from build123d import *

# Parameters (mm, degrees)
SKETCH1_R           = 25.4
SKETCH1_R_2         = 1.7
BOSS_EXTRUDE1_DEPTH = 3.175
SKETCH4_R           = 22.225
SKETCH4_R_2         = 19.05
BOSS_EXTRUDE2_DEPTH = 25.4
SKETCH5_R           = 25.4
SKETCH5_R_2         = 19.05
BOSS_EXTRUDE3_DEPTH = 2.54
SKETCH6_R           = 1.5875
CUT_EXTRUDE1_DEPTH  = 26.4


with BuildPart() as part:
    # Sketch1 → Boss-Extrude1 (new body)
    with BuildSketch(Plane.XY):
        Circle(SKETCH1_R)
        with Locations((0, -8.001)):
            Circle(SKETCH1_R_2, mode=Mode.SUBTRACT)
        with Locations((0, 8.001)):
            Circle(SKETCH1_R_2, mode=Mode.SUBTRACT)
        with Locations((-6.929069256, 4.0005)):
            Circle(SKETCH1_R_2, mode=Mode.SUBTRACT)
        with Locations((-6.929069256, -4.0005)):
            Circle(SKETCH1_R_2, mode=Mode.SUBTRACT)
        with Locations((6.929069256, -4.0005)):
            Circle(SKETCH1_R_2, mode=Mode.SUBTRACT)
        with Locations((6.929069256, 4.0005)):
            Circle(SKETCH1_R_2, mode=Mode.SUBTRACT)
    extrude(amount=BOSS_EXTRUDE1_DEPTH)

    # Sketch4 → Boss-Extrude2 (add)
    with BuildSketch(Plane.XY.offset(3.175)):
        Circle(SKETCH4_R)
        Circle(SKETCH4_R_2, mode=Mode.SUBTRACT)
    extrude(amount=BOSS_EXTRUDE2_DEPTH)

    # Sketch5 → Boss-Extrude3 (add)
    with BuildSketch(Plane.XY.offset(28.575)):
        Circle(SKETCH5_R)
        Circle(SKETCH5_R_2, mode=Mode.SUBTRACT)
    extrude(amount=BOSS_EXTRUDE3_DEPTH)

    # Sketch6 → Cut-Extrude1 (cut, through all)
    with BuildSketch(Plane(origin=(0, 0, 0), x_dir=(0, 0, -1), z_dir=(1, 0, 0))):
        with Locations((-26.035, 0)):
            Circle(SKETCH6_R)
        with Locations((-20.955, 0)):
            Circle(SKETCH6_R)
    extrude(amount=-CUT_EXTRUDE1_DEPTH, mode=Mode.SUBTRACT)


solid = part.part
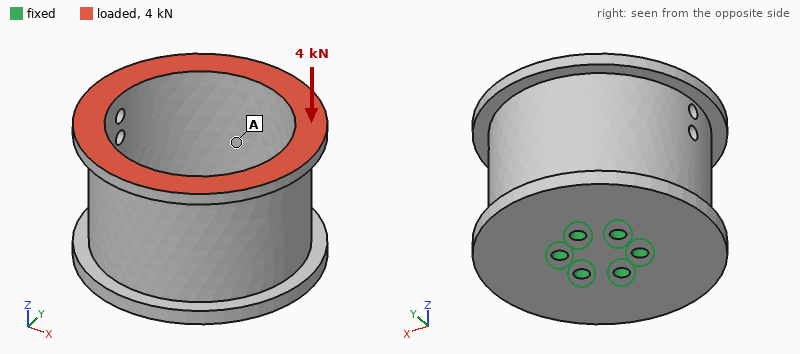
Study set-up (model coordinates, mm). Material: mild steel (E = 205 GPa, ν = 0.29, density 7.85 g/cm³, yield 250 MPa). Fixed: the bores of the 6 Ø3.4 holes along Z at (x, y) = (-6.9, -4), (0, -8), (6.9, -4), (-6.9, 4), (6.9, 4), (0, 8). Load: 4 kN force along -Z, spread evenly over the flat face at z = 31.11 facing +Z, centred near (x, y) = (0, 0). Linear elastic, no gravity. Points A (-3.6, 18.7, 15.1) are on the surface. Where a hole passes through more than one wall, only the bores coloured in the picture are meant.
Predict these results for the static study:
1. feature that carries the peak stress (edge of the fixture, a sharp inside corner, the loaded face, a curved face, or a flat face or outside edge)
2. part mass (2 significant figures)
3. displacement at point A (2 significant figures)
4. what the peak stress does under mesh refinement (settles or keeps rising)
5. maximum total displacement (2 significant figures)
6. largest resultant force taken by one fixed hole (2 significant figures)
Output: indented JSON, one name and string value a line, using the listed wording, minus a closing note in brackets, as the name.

{
  "feature that carries the peak stress": "edge of the fixture",
  "part mass": "150 g",
  "displacement at point A": "17 µm",
  "what the peak stress does under mesh refinement": "keeps rising",
  "maximum total displacement": "20 µm",
  "largest resultant force taken by one fixed hole": "700 N"
}
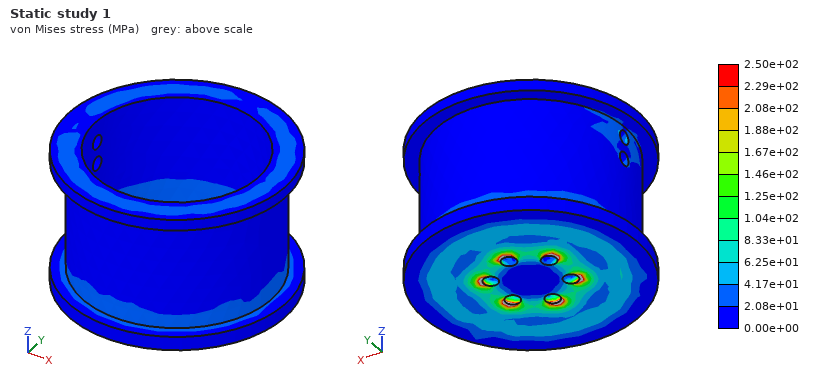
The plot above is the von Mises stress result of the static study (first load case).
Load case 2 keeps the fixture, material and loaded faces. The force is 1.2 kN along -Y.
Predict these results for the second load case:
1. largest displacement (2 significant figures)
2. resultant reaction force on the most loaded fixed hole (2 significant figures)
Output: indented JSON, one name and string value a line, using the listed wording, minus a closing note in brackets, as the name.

{
  "largest displacement": "51 µm",
  "resultant reaction force on the most loaded fixed hole": "810 N"
}
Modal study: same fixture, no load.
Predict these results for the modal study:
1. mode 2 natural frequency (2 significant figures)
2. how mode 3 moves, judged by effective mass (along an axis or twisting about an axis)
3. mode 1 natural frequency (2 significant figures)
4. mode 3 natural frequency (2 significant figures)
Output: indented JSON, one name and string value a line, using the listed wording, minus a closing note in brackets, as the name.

{
  "mode 2 natural frequency": "3300 Hz",
  "how mode 3 moves, judged by effective mass": "along Z",
  "mode 1 natural frequency": "3300 Hz",
  "mode 3 natural frequency": "6900 Hz"
}
